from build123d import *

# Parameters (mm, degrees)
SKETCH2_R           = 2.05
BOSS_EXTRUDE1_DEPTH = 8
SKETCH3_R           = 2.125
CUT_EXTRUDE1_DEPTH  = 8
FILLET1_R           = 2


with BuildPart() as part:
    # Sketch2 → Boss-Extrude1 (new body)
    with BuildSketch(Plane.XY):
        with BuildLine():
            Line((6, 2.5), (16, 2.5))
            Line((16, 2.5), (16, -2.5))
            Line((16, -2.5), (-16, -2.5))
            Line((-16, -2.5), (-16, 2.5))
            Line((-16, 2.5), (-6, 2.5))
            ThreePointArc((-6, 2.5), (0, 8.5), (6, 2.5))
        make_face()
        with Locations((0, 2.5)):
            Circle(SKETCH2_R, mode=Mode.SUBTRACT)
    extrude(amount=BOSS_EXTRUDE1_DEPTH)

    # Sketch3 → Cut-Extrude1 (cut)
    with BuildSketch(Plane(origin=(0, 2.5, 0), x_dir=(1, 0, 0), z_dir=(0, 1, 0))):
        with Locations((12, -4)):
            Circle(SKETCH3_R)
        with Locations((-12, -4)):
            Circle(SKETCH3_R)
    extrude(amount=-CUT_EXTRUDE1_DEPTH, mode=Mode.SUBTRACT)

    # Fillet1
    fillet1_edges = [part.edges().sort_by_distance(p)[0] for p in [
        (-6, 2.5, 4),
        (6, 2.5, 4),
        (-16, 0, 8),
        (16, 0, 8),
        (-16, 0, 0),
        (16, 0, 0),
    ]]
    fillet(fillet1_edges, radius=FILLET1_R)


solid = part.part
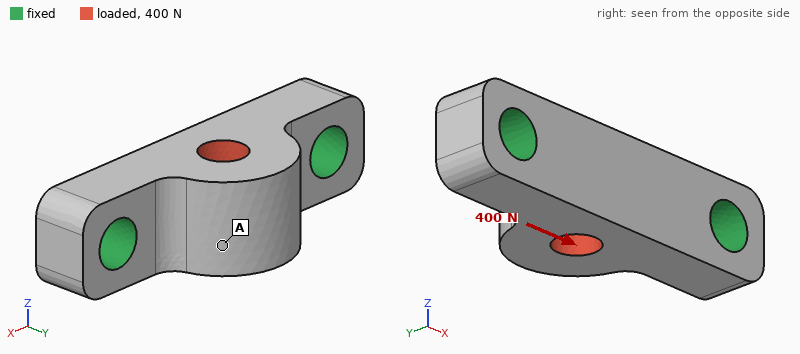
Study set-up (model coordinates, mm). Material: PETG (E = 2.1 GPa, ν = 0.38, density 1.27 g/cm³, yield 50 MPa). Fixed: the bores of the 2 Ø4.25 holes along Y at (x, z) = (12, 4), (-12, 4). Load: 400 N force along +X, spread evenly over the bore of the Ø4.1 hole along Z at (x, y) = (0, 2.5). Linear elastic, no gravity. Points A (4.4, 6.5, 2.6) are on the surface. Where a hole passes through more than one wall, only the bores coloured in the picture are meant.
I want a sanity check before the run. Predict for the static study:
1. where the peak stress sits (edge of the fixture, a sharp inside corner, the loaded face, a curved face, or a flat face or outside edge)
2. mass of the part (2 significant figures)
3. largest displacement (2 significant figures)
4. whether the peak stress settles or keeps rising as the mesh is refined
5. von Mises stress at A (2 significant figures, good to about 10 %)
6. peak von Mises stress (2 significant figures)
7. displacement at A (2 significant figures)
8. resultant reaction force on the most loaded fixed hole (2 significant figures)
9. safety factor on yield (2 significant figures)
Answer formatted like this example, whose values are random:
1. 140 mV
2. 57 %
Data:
1. a curved face
2. 1.9 g
3. 37 µm
4. settles
5. 2.0 MPa
6. 15 MPa
7. 33 µm
8. 210 N
9. 3.4
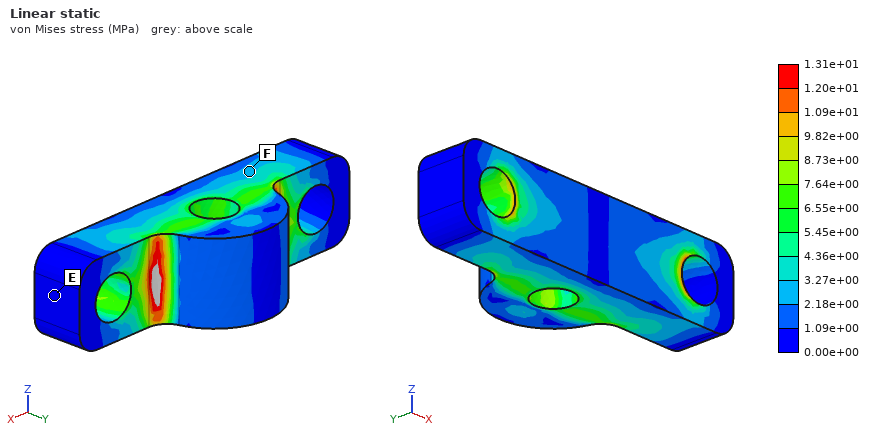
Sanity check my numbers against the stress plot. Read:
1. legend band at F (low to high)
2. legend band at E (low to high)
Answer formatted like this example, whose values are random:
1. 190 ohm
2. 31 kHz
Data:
1. 2.18e+00 to 3.27e+00 MPa
2. 0.00e+00 to 1.09e+00 MPa
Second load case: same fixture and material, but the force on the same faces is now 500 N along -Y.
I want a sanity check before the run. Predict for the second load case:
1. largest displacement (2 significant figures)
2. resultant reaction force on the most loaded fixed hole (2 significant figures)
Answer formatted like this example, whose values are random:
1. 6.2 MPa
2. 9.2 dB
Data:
1. 0.13 mm
2. 260 N
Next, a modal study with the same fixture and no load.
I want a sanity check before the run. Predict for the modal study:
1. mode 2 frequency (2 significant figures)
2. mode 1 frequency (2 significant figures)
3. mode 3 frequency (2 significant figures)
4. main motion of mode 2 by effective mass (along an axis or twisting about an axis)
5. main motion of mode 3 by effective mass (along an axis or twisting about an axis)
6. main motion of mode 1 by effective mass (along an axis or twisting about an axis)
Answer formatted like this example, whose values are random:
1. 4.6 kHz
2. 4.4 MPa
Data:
1. 11 kHz
2. 7100 Hz
3. 13 kHz
4. along Y
5. along Z
6. along Z
